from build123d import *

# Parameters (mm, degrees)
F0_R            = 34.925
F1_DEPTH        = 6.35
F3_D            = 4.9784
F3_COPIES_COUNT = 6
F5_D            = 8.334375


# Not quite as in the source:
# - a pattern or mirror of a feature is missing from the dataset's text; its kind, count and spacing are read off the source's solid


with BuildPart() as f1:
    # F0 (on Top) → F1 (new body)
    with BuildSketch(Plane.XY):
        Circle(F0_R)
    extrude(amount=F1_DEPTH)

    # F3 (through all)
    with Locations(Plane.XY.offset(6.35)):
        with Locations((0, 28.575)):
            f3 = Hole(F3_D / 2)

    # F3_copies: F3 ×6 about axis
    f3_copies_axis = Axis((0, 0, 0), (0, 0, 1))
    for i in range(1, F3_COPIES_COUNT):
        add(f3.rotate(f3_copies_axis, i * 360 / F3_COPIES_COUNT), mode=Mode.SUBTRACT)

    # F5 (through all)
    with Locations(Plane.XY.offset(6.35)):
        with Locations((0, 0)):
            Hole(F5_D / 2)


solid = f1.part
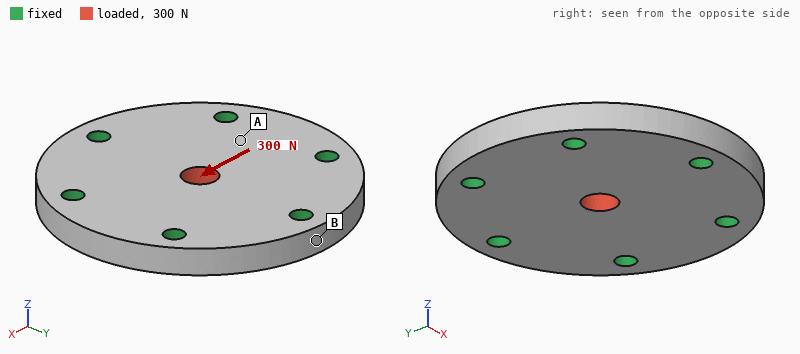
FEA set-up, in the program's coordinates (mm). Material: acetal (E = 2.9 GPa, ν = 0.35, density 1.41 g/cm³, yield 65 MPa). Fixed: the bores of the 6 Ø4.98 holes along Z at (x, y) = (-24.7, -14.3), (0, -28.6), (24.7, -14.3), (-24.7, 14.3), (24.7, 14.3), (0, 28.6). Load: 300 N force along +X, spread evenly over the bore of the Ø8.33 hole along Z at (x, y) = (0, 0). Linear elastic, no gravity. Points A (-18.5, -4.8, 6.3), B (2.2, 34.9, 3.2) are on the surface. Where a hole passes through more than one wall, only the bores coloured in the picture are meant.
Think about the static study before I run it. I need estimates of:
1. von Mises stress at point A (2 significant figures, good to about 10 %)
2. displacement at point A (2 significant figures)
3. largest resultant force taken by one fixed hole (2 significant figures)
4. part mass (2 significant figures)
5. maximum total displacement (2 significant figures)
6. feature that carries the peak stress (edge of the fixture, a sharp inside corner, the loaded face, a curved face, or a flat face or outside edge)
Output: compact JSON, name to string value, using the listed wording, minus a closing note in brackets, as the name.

{"von Mises stress at point A": "0.64 MPa", "displacement at point A": "3.4 µm", "largest resultant force taken by one fixed hole": "70 N", "part mass": "33 g", "maximum total displacement": "9.4 µm", "feature that carries the peak stress": "the loaded face"}
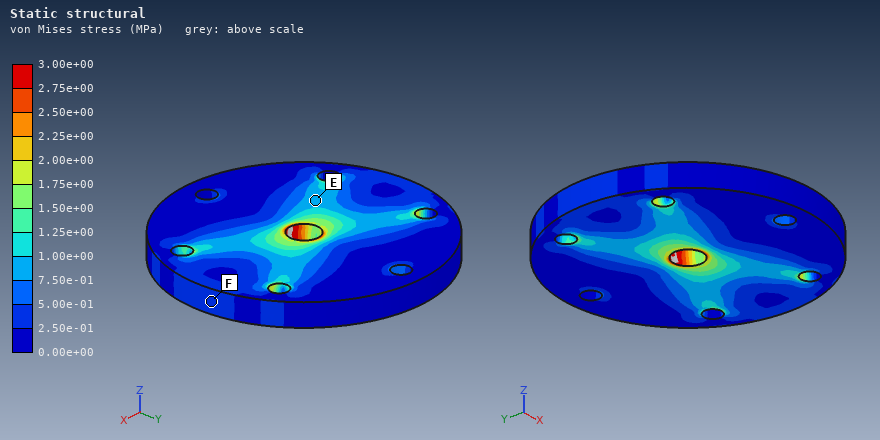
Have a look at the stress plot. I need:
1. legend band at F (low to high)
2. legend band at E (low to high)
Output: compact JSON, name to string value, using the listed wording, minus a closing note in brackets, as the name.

{"legend band at F": "2.50e-01 to 5.00e-01 MPa", "legend band at E": "7.50e-01 to 1.00e+00 MPa"}
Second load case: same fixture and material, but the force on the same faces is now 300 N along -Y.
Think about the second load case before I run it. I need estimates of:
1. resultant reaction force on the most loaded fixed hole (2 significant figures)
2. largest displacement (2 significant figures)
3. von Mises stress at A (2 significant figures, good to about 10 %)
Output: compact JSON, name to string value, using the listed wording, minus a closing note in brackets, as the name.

{"resultant reaction force on the most loaded fixed hole": "79 N", "largest displacement": "9.4 µm", "von Mises stress at A": "0.36 MPa"}
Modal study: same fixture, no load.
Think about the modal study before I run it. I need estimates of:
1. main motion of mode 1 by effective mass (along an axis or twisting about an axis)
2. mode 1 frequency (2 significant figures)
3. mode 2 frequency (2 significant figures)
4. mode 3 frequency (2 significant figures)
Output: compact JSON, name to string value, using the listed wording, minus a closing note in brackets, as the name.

{"main motion of mode 1 by effective mass": "along Z", "mode 1 frequency": "4400 Hz", "mode 2 frequency": "8100 Hz", "mode 3 frequency": "8100 Hz"}
